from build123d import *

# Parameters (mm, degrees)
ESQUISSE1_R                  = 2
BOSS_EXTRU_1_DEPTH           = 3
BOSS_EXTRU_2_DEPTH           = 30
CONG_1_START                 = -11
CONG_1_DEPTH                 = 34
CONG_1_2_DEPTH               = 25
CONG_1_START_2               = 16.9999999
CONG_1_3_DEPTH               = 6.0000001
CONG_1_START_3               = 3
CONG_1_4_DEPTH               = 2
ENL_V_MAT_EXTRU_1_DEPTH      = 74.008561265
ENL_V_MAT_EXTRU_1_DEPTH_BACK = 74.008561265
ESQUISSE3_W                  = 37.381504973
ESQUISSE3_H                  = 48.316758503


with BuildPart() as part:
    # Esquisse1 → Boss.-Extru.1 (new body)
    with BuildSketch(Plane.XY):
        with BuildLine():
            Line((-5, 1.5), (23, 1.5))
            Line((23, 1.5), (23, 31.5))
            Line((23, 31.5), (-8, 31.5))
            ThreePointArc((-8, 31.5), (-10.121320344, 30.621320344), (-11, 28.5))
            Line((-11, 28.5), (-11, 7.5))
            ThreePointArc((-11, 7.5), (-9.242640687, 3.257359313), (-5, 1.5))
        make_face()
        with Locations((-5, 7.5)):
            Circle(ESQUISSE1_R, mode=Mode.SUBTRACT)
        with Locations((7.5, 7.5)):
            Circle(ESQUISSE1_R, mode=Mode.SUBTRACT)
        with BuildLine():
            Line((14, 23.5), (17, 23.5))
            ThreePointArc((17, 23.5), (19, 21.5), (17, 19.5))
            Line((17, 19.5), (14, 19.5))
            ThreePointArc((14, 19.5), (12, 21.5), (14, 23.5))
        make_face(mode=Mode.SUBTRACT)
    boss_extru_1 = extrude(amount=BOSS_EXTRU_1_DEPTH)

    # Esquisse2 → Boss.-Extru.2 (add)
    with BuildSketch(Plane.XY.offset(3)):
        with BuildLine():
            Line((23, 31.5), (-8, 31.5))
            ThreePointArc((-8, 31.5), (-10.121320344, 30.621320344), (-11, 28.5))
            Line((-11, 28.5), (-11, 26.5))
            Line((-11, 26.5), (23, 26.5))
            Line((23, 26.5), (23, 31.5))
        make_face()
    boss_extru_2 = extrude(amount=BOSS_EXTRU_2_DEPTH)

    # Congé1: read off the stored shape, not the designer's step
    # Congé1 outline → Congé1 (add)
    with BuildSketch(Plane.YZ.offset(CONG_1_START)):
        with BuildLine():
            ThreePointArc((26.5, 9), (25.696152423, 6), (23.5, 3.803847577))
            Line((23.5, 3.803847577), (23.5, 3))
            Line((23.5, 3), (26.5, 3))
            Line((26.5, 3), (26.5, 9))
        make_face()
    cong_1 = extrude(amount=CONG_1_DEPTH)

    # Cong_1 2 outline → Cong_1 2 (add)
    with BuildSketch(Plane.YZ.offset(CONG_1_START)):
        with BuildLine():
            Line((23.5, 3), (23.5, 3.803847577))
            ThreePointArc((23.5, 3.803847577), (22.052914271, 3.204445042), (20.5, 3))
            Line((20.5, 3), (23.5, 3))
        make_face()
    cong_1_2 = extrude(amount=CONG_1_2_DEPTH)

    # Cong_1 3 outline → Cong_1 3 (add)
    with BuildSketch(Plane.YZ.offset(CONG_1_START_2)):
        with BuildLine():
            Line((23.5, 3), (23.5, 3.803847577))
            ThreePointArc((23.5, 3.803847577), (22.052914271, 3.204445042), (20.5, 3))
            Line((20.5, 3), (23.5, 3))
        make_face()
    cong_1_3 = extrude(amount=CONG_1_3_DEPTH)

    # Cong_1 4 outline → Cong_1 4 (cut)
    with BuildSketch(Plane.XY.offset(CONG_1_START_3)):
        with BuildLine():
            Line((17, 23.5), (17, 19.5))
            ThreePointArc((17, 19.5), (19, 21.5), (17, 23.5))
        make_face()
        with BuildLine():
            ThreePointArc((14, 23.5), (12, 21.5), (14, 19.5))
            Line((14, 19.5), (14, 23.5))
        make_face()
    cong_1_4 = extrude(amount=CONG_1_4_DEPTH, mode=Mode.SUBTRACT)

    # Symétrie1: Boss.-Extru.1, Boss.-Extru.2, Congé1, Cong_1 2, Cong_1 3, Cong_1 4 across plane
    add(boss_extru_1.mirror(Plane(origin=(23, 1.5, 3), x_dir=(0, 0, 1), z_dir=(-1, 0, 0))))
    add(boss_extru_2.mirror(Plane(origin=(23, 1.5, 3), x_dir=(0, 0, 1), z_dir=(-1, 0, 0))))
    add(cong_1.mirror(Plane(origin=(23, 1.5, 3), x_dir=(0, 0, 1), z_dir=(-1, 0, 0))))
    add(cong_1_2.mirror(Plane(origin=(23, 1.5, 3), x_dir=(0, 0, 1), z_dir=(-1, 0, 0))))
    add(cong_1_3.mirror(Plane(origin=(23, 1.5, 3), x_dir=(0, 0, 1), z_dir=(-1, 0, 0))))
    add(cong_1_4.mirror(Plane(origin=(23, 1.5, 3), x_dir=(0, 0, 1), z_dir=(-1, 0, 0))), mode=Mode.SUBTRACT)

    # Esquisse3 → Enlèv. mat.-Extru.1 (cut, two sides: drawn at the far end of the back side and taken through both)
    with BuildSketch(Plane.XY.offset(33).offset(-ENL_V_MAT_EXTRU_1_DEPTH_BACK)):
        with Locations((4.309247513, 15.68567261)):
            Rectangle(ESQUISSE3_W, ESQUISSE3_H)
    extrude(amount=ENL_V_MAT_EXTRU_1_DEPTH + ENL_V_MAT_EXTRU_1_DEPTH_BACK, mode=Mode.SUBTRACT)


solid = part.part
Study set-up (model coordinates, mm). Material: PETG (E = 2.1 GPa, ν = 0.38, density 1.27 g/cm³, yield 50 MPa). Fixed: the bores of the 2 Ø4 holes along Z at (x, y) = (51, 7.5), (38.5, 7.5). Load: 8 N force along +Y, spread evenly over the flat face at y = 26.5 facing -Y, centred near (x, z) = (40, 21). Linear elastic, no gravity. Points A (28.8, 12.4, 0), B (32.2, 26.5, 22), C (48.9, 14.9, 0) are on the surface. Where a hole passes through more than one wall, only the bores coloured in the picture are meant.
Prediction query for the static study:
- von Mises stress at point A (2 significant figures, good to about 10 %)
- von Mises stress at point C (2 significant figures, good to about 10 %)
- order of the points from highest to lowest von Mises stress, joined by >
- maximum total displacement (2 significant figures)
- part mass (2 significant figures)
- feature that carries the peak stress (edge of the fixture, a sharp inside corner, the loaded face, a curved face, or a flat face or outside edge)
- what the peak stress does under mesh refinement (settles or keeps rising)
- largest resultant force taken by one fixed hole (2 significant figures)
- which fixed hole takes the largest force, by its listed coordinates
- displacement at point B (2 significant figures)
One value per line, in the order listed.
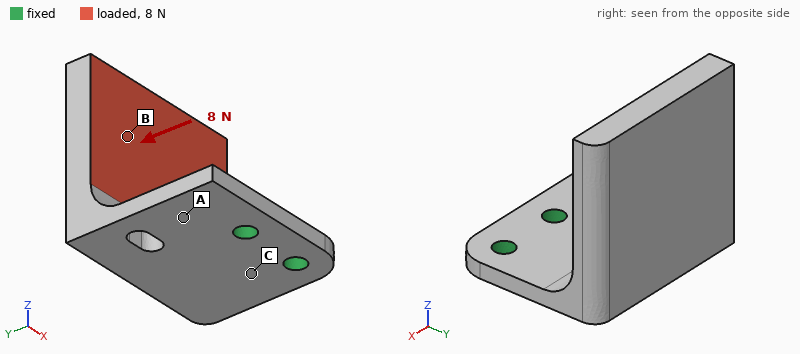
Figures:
1.9 MPa
3.1 MPa
C > A > B
0.61 mm
10 g
edge of the fixture
keeps rising
6.6 N
(38.5, 7.5)
0.39 mm
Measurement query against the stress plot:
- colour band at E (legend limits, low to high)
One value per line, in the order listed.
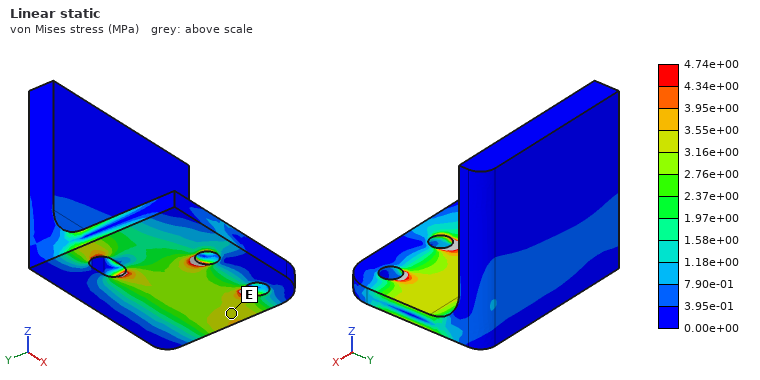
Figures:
3.16e+00 to 3.55e+00 MPa
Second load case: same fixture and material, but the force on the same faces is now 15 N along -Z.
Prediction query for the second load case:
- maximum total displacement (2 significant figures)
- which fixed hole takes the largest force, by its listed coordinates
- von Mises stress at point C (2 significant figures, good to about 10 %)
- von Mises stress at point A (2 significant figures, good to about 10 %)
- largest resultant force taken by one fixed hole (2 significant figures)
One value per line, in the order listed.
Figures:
0.59 mm
(38.5, 7.5)
3.5 MPa
2.4 MPa
11 N
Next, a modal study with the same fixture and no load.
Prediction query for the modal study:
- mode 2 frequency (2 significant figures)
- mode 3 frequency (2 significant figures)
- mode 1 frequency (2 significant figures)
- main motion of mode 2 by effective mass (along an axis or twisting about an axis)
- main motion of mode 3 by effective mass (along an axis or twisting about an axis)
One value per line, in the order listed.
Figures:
480 Hz
1100 Hz
260 Hz
along X
along Z
